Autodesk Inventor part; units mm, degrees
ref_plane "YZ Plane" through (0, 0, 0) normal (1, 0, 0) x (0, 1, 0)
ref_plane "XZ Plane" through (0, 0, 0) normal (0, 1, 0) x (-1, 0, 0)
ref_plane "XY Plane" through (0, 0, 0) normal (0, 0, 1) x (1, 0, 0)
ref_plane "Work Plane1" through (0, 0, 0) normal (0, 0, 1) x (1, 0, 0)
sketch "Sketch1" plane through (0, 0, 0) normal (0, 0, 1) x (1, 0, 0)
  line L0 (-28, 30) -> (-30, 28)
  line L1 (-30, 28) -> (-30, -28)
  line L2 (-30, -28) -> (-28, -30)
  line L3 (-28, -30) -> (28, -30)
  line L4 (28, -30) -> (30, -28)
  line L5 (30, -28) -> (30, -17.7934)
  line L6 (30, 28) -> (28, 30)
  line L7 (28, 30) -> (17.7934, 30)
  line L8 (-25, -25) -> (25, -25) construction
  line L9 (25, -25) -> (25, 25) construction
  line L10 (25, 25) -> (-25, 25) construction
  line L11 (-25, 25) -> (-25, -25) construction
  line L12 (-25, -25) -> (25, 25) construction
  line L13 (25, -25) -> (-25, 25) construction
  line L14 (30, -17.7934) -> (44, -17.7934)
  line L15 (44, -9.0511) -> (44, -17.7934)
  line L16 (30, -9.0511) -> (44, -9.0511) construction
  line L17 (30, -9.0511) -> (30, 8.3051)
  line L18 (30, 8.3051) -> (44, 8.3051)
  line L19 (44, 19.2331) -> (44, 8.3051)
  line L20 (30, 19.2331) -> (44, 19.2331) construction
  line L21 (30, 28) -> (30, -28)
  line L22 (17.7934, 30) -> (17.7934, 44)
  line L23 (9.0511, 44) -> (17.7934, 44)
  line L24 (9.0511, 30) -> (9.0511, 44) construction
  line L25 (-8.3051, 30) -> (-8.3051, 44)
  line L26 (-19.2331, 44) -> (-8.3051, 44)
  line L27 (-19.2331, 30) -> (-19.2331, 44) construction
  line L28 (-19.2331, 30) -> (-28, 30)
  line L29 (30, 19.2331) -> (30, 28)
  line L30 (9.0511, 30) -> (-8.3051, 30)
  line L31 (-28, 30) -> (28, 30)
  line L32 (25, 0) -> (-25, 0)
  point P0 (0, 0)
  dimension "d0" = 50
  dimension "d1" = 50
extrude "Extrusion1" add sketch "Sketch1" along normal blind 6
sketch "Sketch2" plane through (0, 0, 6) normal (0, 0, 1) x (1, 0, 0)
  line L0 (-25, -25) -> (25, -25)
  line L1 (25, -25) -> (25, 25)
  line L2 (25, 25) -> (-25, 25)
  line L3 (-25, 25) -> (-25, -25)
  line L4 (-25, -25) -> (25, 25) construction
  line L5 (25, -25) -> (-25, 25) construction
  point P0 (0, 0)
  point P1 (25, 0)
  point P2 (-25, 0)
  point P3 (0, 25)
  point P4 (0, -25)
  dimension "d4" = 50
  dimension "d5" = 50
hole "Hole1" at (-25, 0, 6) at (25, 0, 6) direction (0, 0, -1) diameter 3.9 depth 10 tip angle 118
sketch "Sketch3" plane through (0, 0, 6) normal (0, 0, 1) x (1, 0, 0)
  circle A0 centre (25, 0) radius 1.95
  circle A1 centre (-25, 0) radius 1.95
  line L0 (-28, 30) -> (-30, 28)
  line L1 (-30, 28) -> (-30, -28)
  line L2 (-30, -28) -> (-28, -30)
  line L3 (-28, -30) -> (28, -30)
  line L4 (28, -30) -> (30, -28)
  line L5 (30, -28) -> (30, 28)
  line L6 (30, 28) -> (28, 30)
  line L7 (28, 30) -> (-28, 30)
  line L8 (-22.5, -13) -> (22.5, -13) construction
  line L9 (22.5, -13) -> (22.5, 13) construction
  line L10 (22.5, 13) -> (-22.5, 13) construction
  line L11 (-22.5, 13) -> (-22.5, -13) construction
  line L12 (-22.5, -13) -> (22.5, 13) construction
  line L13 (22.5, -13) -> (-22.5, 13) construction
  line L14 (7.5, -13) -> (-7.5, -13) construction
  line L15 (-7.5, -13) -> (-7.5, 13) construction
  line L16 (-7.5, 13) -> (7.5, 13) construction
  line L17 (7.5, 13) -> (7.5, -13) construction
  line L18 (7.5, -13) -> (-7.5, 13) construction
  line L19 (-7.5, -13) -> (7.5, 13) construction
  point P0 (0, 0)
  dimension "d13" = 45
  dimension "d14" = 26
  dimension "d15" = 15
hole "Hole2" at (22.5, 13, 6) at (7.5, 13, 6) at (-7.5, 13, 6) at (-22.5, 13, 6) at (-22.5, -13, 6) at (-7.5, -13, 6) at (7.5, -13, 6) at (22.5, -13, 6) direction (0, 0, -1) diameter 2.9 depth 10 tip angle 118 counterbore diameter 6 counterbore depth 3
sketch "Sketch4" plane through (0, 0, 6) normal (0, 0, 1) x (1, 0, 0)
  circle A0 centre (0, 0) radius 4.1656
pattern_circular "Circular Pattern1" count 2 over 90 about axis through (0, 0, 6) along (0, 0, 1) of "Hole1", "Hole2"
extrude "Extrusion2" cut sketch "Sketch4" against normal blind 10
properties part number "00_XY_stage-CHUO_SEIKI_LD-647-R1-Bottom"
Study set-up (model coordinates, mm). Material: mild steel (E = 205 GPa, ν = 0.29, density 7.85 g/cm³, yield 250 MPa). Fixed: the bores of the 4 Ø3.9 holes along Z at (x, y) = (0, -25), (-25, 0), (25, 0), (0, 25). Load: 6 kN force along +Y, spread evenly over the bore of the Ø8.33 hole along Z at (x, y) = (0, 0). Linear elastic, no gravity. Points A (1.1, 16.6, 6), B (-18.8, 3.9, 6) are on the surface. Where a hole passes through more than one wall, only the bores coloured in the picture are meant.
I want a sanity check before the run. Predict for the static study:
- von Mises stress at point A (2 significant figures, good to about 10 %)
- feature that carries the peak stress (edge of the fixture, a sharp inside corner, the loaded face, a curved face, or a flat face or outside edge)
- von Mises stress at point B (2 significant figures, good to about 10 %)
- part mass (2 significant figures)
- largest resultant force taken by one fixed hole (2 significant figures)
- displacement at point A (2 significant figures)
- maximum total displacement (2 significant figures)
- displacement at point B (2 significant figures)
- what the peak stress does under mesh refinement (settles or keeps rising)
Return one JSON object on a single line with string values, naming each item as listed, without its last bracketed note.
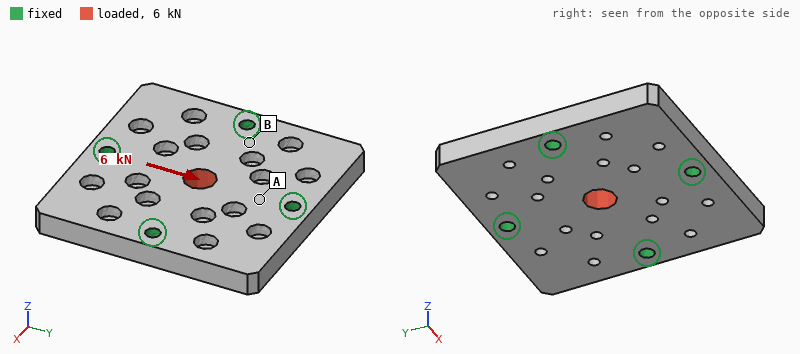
{"von Mises stress at point A": "33 MPa", "feature that carries the peak stress": "edge of the fixture", "von Mises stress at point B": "7.2 MPa", "part mass": "150 g", "largest resultant force taken by one fixed hole": "2.0 kN", "displacement at point A": "1.1 µm", "maximum total displacement": "3.4 µm", "displacement at point B": "0.75 µm", "what the peak stress does under mesh refinement": "keeps rising"}
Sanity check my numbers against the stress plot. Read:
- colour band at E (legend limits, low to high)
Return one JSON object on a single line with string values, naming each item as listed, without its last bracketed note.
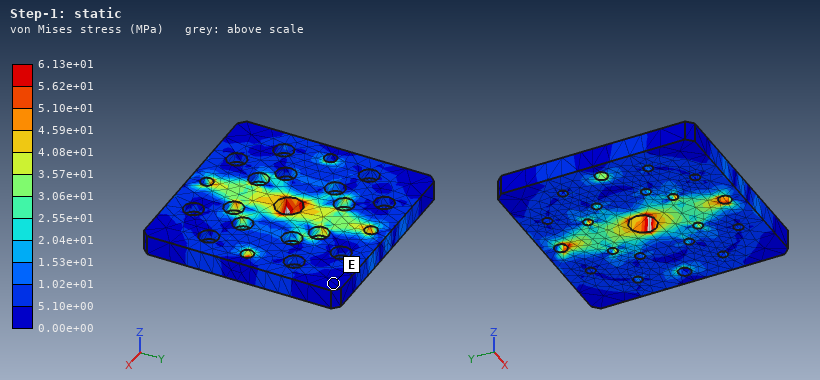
{"colour band at E": "0.00e+00 to 5.10e+00 MPa"}
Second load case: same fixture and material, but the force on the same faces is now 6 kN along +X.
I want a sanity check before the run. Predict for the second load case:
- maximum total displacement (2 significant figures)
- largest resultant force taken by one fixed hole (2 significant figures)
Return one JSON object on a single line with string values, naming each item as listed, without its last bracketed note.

{"maximum total displacement": "3.4 µm", "largest resultant force taken by one fixed hole": "2.0 kN"}
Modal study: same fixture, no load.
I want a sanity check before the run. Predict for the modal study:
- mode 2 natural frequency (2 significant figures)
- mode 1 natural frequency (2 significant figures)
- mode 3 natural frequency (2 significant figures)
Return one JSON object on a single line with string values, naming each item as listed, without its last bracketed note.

{"mode 2 natural frequency": "10 kHz", "mode 1 natural frequency": "9700 Hz", "mode 3 natural frequency": "10 kHz"}
